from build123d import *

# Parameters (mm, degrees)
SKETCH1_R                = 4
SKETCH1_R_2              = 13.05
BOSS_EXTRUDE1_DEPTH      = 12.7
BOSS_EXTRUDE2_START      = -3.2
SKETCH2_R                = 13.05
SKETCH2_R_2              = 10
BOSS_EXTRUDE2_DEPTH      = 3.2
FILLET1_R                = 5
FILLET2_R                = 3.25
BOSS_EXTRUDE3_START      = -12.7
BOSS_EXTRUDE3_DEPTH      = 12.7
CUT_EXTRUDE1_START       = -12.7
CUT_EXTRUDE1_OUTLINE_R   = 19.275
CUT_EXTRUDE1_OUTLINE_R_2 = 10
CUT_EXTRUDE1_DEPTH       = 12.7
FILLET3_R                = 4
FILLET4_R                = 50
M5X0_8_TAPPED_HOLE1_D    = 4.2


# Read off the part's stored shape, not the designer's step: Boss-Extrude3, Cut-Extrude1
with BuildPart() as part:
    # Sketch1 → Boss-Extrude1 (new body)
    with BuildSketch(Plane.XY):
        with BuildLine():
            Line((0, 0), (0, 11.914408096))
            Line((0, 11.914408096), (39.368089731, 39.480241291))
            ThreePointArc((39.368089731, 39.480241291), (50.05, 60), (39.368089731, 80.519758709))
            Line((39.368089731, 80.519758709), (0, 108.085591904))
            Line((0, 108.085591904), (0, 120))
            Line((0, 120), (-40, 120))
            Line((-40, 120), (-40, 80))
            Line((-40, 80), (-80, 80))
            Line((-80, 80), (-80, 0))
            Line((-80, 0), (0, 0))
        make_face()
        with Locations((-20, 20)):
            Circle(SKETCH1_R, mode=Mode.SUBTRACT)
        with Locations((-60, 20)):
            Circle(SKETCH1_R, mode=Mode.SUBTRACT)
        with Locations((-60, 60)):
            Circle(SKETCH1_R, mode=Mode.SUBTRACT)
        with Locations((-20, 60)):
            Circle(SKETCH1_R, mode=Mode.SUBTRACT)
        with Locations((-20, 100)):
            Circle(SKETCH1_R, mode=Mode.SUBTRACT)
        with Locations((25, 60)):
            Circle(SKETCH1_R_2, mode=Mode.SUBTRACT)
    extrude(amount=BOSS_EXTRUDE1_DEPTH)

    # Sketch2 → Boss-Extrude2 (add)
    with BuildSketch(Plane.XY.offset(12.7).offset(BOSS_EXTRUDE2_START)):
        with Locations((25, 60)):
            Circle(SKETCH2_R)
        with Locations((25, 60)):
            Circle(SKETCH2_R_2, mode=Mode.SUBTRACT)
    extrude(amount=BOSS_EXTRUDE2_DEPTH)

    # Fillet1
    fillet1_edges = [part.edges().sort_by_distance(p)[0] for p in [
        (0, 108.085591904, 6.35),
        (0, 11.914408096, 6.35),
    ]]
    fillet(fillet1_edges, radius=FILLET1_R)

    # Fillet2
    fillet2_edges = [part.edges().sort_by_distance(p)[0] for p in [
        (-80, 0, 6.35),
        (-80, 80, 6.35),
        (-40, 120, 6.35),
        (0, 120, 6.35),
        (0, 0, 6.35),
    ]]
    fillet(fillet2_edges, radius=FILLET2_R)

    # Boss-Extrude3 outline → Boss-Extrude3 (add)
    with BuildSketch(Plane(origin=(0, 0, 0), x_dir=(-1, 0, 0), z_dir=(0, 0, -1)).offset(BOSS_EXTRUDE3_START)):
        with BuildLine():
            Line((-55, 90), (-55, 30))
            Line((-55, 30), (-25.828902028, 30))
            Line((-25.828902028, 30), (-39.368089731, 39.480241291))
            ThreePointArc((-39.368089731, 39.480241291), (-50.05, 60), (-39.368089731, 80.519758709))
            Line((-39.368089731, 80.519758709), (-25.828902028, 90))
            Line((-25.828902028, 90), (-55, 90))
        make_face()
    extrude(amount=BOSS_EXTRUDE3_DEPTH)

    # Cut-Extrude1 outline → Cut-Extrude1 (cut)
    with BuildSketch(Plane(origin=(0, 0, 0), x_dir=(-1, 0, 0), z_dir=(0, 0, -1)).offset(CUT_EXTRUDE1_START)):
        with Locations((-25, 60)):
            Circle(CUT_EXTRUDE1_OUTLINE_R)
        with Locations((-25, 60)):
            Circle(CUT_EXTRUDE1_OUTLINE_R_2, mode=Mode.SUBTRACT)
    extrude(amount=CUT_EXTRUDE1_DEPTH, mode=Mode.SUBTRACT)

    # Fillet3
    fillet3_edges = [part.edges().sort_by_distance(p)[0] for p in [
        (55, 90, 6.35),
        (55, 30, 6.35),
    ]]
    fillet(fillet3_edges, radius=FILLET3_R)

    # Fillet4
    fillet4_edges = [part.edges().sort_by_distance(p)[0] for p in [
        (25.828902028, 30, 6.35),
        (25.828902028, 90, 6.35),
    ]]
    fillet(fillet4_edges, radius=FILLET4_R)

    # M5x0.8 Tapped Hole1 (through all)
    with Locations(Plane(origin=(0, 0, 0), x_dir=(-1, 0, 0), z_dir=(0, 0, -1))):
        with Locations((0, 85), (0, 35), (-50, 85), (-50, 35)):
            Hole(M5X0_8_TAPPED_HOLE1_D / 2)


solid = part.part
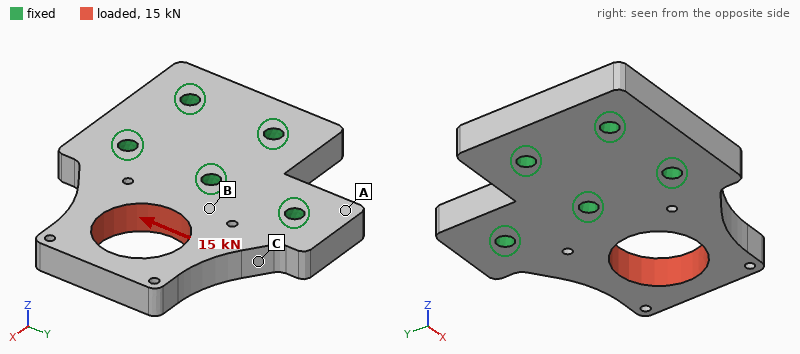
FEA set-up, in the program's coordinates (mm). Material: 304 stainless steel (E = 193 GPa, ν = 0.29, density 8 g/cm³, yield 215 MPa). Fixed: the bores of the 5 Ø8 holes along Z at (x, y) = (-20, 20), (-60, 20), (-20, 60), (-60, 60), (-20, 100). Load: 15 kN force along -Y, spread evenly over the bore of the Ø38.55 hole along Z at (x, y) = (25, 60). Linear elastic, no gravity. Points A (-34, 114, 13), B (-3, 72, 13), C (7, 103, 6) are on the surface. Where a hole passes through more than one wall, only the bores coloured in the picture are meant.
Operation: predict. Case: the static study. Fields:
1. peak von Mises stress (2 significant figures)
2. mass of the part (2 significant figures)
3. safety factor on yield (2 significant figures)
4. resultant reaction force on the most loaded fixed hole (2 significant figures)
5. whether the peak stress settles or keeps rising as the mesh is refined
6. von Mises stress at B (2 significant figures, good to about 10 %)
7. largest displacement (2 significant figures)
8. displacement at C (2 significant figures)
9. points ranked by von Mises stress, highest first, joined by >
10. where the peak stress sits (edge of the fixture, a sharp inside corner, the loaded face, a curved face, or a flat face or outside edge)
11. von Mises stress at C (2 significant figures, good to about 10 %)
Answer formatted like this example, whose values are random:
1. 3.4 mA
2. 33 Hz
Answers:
1. 84 MPa
2. 1.0 kg
3. 2.6
4. 8.9 kN
5. settles
6. 33 MPa
7. 35 µm
8. 6.9 µm
9. C > B > A
10. the loaded face
11. 47 MPa
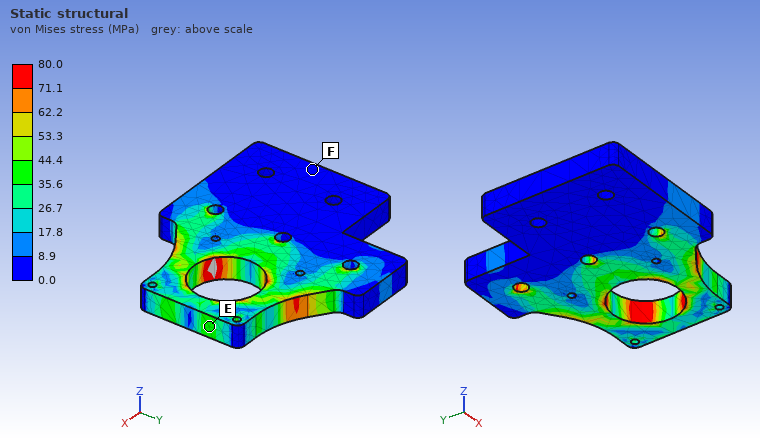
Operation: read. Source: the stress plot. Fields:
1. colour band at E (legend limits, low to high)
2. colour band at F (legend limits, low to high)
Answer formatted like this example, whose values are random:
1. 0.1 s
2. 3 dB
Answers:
1. 35.6 to 44.4 MPa
2. 0.0 to 8.9 MPa
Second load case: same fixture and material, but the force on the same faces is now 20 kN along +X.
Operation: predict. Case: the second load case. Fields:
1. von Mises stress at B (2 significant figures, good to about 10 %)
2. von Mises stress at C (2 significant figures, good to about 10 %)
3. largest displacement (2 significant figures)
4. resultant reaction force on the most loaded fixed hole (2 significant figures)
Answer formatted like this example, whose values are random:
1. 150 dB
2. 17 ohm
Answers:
1. 15 MPa
2. 19 MPa
3. 16 µm
4. 6.6 kN
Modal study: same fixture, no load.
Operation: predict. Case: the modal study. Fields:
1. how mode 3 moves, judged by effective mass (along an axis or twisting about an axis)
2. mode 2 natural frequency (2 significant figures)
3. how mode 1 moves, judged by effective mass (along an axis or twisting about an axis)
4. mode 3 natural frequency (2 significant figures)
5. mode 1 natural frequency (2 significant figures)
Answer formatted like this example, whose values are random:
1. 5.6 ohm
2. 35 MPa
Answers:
1. along Y
2. 4800 Hz
3. along Z
4. 7200 Hz
5. 2200 Hz
